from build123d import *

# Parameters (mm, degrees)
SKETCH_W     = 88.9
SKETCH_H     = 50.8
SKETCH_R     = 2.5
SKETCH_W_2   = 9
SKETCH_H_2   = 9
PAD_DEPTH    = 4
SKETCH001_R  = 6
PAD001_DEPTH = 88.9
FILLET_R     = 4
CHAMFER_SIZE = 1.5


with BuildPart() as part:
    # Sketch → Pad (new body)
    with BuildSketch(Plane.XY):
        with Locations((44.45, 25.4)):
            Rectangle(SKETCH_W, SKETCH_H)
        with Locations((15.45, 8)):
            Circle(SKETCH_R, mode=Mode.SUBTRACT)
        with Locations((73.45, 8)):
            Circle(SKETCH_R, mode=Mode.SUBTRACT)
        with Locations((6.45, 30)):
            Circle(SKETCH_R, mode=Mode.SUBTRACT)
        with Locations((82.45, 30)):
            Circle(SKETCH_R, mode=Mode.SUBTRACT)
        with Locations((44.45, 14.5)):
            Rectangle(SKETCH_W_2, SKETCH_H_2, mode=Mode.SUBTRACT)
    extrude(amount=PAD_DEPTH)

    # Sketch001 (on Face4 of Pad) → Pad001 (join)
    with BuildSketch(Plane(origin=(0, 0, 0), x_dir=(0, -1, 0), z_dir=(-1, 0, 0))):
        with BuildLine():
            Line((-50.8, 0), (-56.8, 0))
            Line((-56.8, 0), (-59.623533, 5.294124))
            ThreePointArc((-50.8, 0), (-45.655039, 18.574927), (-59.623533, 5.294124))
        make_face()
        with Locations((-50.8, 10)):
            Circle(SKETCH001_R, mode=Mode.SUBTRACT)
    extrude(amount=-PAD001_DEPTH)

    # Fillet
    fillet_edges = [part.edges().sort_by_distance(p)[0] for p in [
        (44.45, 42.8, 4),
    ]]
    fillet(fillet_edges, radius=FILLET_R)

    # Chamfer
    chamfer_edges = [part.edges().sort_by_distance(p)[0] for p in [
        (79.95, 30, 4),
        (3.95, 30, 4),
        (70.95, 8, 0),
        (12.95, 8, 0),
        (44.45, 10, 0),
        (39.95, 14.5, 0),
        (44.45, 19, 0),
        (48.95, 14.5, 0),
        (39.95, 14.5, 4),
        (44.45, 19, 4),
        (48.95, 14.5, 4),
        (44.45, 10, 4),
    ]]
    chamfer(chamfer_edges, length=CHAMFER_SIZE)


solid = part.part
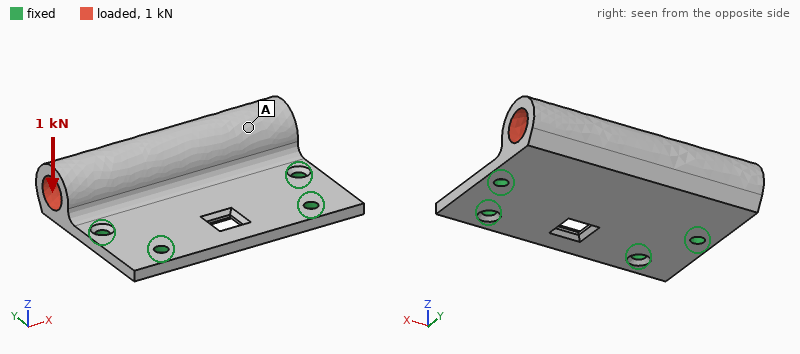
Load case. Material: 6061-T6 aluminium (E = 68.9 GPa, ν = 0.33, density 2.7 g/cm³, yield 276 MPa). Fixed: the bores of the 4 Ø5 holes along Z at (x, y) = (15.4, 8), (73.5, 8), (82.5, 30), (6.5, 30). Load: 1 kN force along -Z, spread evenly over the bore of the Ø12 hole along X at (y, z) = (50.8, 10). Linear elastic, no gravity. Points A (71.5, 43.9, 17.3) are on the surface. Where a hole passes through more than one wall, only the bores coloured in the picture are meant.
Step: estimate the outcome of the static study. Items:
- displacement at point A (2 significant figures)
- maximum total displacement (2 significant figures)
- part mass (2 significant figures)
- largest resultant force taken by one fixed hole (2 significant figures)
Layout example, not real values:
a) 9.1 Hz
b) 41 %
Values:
a) 0.14 mm
b) 0.22 mm
c) 92 g
d) 840 N
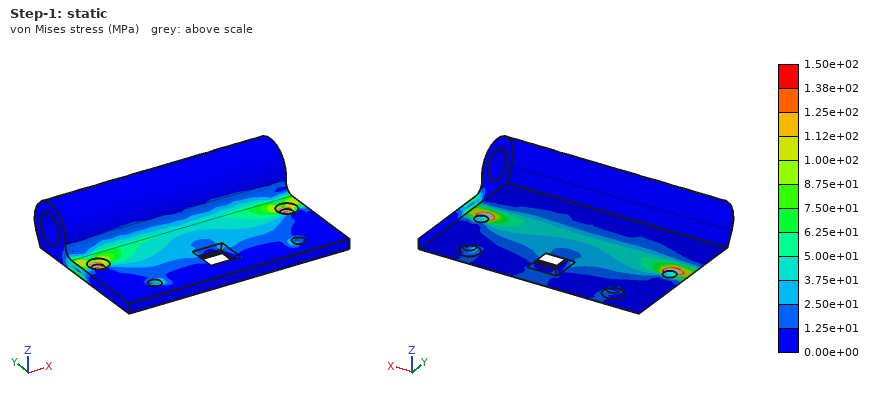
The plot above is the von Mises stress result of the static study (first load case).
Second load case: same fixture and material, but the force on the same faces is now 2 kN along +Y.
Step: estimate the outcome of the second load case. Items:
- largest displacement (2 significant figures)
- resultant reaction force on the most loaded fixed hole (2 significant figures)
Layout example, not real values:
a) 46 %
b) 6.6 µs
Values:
a) 0.21 mm
b) 630 N
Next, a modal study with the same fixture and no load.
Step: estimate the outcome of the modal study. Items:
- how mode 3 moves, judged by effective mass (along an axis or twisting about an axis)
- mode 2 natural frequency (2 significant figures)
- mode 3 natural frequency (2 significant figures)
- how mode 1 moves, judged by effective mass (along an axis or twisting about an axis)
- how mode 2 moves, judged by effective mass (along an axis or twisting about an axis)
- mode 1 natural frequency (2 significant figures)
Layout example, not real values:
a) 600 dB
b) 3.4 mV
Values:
a) along Z
b) 5800 Hz
c) 6100 Hz
d) along Z
e) twisting about Y
f) 1600 Hz
